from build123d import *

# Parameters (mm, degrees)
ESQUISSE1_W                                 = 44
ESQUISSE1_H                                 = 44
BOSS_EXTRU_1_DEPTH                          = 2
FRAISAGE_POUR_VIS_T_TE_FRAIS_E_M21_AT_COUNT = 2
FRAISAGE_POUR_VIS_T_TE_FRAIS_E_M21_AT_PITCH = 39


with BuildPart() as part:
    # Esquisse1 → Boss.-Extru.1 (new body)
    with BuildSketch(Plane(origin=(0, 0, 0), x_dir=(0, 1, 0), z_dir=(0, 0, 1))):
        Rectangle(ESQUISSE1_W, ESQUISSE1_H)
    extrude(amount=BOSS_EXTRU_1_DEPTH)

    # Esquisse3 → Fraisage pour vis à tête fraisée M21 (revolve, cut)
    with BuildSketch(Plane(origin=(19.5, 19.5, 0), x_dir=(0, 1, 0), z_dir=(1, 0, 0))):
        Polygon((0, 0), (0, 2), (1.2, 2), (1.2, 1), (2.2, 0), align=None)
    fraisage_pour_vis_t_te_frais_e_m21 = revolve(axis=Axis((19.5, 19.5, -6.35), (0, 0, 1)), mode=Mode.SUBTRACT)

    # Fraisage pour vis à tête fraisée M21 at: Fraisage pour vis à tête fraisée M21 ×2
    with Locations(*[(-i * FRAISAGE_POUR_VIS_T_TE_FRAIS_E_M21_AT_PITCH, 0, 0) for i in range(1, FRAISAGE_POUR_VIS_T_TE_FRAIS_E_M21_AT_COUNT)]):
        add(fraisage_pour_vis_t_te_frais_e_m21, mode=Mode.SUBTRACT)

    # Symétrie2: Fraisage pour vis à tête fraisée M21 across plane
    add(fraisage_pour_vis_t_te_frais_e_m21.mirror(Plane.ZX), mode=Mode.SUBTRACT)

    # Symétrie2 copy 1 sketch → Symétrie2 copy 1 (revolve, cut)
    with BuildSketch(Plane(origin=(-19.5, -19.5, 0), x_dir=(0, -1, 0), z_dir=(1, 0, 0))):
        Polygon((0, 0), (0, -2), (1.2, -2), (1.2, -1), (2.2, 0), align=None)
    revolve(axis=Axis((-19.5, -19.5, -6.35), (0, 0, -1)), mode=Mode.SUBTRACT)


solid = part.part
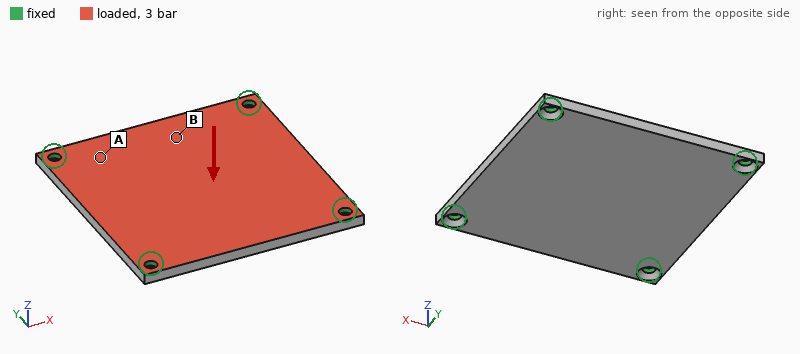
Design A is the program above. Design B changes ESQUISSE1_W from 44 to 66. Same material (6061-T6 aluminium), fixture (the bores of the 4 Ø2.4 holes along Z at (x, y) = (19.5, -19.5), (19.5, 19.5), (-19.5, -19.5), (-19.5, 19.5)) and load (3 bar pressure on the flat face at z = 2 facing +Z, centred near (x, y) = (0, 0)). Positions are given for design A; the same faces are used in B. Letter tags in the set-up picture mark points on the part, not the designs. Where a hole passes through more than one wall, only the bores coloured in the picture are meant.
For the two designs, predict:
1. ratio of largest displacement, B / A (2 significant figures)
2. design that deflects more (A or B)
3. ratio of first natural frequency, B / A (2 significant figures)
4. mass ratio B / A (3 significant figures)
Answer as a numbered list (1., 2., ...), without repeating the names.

1. 0.85
2. A
3. 1.0
4. 1.51
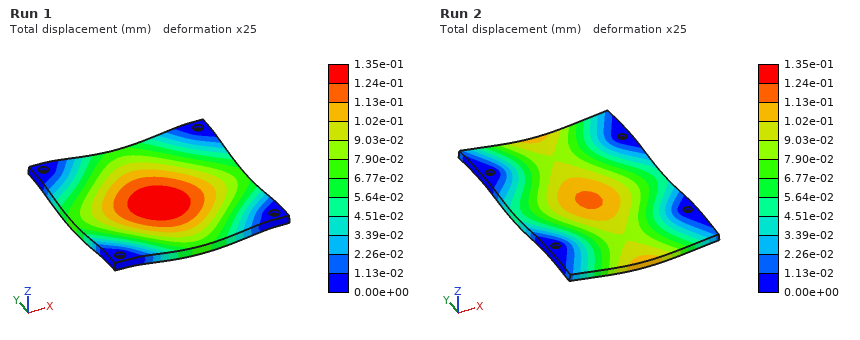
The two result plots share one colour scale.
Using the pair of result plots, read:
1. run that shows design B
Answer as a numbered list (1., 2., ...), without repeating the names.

1. Run 2
